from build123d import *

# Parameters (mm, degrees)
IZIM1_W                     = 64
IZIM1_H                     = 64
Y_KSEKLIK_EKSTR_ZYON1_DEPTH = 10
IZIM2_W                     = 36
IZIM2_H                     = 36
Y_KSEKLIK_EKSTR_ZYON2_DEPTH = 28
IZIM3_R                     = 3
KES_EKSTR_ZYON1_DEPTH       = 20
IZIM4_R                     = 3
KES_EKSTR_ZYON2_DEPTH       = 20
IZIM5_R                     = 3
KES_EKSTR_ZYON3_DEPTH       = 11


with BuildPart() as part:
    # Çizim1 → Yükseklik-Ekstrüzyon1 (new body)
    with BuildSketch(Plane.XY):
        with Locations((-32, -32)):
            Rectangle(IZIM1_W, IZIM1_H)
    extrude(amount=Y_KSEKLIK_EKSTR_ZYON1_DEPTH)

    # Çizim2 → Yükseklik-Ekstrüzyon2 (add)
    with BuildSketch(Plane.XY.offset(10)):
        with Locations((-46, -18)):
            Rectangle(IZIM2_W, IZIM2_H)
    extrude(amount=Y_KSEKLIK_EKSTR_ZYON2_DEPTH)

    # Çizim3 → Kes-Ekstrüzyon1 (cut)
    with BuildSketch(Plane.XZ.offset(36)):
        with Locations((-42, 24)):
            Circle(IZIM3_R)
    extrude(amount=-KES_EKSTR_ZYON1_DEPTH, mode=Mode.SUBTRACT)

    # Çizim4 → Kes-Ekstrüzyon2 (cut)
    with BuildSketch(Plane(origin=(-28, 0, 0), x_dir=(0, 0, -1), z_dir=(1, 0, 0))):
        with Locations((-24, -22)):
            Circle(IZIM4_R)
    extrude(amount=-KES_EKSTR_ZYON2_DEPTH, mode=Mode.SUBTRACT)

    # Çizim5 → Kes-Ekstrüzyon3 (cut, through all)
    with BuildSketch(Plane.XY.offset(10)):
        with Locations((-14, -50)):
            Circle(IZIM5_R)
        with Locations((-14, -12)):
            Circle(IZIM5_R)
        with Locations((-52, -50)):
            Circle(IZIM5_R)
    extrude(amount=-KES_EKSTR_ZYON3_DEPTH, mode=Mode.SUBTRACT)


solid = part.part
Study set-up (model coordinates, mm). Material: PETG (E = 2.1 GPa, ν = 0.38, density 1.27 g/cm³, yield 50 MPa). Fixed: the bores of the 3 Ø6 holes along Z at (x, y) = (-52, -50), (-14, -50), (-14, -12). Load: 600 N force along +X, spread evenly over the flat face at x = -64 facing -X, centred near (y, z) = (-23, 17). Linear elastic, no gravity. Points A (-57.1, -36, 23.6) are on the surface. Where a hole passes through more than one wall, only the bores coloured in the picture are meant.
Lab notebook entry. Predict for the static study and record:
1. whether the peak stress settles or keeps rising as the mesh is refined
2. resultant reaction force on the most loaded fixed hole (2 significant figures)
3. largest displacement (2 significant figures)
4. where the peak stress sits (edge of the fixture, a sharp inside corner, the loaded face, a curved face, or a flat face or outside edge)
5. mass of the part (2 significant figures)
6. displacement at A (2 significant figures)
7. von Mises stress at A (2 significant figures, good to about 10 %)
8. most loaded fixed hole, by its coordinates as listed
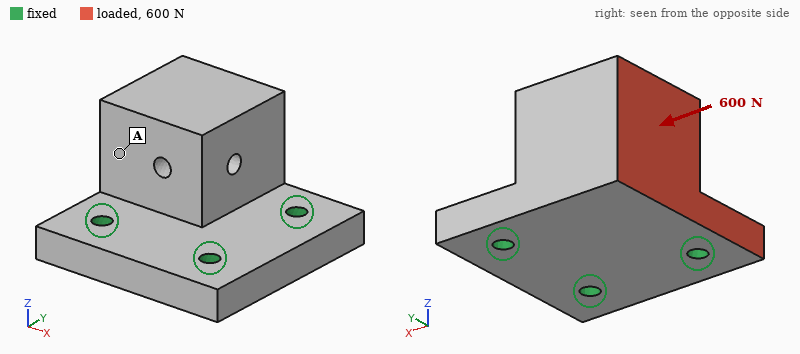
keeps rising
310 N
0.24 mm
edge of the fixture
96 g
0.11 mm
0.78 MPa
(-14, -12)
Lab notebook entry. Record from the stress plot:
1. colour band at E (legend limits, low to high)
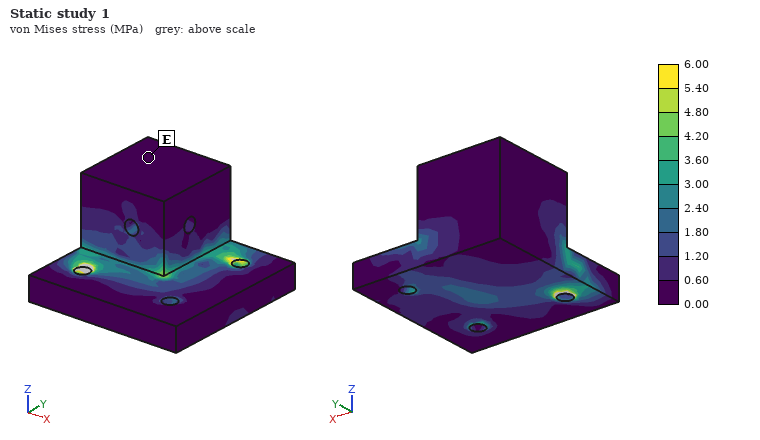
0.00 to 0.60 MPa
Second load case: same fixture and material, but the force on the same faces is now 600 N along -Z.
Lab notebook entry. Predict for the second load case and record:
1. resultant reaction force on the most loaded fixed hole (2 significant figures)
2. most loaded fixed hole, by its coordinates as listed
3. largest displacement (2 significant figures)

610 N
(-52, -50)
0.70 mm
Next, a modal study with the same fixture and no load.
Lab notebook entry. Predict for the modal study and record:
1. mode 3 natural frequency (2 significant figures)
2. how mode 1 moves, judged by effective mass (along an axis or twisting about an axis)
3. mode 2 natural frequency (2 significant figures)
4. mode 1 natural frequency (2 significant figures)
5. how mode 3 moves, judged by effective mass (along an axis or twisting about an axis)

2600 Hz
along Z
1900 Hz
820 Hz
along Z
